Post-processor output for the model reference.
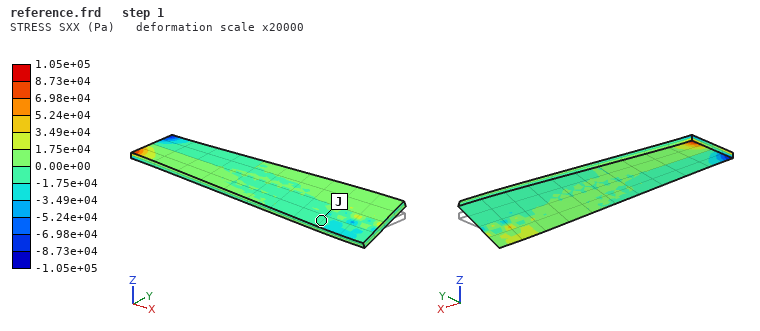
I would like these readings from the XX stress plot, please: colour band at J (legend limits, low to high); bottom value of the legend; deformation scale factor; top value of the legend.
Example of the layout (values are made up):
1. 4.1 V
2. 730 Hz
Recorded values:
1. -1.75e+04 to 0.00e+00 Pa
2. -1.05e+05 Pa
3. 20000
4. 1.05e+05 Pa
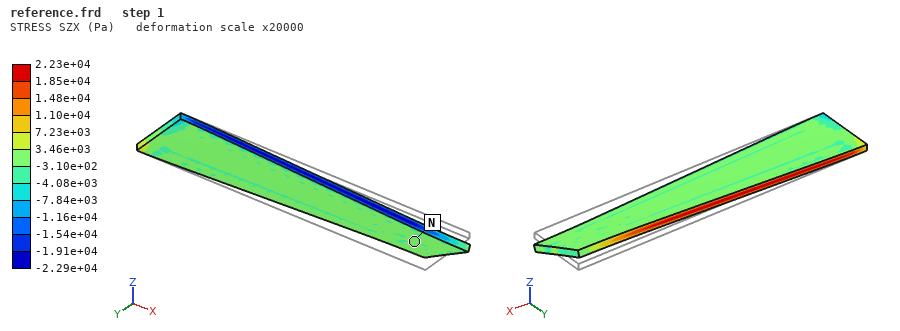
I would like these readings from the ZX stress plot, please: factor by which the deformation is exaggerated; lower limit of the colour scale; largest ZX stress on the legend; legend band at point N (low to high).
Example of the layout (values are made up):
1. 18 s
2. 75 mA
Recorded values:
1. 20000
2. -2.29e+04 Pa
3. 2.23e+04 Pa
4. -3.10e+02 to 3.46e+03 Pa
